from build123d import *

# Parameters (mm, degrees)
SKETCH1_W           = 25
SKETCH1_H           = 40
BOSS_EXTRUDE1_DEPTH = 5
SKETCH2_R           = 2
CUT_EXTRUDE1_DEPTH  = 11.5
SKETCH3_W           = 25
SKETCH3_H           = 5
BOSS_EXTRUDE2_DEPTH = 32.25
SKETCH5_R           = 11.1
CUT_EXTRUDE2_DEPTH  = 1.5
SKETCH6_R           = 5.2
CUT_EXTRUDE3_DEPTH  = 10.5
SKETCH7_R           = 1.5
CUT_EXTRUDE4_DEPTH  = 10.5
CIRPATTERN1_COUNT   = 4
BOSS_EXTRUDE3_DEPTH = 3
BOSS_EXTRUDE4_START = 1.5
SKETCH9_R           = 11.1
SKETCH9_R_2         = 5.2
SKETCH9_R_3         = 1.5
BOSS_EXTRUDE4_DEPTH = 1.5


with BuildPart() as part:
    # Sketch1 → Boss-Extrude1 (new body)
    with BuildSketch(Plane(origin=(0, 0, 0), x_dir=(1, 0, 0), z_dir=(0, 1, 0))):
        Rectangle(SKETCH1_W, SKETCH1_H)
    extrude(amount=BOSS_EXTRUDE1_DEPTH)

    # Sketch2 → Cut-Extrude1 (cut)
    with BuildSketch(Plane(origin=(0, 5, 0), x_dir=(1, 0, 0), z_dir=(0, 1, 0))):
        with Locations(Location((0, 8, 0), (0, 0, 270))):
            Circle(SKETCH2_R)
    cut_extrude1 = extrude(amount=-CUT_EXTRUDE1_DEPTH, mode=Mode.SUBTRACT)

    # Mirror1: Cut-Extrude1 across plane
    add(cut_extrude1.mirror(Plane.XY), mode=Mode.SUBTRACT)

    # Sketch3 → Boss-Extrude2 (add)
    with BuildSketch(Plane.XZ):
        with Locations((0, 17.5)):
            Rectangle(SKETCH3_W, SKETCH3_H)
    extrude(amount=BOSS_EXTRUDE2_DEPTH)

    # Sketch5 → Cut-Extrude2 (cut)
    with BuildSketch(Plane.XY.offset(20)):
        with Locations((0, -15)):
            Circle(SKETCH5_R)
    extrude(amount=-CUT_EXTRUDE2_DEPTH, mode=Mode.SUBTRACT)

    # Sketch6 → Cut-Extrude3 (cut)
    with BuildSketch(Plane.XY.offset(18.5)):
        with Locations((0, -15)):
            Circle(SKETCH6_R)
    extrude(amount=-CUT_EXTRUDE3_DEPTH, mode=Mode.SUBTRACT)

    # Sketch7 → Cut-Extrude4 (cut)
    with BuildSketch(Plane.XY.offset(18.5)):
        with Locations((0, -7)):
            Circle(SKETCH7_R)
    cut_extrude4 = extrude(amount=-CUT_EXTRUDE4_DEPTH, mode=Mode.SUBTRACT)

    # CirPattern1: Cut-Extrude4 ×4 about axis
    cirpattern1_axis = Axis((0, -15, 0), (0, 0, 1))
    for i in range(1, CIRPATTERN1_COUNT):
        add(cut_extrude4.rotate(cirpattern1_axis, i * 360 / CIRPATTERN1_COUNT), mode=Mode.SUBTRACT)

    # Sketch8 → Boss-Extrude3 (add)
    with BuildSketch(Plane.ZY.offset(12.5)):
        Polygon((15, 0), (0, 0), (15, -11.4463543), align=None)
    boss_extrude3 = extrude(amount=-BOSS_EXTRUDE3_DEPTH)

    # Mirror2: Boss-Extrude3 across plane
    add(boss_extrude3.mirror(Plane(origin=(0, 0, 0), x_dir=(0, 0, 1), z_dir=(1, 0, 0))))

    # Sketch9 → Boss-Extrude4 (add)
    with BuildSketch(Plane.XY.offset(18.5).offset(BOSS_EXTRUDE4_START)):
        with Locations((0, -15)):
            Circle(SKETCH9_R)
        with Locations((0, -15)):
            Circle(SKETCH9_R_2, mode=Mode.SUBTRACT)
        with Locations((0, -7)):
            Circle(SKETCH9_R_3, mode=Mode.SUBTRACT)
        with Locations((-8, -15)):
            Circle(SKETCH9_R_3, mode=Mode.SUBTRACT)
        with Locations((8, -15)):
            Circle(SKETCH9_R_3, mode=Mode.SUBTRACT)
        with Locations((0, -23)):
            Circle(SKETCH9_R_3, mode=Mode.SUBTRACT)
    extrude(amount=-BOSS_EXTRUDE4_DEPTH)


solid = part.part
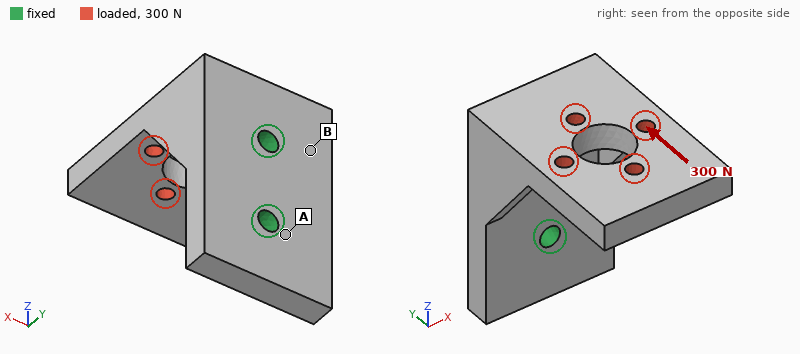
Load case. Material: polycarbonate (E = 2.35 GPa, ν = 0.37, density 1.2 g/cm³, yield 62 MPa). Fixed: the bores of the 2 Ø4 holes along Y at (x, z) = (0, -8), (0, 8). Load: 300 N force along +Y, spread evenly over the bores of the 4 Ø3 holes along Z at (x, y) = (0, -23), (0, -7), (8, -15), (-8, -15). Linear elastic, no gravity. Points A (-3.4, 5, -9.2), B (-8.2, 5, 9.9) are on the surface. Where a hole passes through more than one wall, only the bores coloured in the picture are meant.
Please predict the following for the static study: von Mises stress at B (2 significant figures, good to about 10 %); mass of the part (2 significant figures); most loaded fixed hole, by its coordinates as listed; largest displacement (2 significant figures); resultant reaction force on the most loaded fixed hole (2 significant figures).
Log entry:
6.0 MPa
11 g
(0, 8)
0.54 mm
370 N
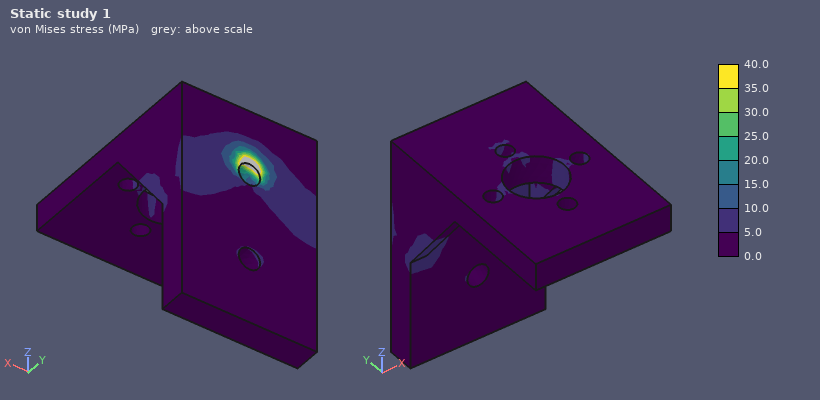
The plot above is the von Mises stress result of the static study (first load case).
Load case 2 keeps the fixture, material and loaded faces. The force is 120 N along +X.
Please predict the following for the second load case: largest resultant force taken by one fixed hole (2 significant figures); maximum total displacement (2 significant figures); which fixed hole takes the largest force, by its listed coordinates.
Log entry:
170 N
0.70 mm
(0, 8)
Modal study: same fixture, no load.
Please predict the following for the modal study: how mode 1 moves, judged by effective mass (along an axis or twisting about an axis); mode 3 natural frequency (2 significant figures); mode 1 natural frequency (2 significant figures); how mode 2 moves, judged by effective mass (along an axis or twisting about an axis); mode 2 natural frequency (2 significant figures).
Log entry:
along Z
2800 Hz
970 Hz
along X
1100 Hz
